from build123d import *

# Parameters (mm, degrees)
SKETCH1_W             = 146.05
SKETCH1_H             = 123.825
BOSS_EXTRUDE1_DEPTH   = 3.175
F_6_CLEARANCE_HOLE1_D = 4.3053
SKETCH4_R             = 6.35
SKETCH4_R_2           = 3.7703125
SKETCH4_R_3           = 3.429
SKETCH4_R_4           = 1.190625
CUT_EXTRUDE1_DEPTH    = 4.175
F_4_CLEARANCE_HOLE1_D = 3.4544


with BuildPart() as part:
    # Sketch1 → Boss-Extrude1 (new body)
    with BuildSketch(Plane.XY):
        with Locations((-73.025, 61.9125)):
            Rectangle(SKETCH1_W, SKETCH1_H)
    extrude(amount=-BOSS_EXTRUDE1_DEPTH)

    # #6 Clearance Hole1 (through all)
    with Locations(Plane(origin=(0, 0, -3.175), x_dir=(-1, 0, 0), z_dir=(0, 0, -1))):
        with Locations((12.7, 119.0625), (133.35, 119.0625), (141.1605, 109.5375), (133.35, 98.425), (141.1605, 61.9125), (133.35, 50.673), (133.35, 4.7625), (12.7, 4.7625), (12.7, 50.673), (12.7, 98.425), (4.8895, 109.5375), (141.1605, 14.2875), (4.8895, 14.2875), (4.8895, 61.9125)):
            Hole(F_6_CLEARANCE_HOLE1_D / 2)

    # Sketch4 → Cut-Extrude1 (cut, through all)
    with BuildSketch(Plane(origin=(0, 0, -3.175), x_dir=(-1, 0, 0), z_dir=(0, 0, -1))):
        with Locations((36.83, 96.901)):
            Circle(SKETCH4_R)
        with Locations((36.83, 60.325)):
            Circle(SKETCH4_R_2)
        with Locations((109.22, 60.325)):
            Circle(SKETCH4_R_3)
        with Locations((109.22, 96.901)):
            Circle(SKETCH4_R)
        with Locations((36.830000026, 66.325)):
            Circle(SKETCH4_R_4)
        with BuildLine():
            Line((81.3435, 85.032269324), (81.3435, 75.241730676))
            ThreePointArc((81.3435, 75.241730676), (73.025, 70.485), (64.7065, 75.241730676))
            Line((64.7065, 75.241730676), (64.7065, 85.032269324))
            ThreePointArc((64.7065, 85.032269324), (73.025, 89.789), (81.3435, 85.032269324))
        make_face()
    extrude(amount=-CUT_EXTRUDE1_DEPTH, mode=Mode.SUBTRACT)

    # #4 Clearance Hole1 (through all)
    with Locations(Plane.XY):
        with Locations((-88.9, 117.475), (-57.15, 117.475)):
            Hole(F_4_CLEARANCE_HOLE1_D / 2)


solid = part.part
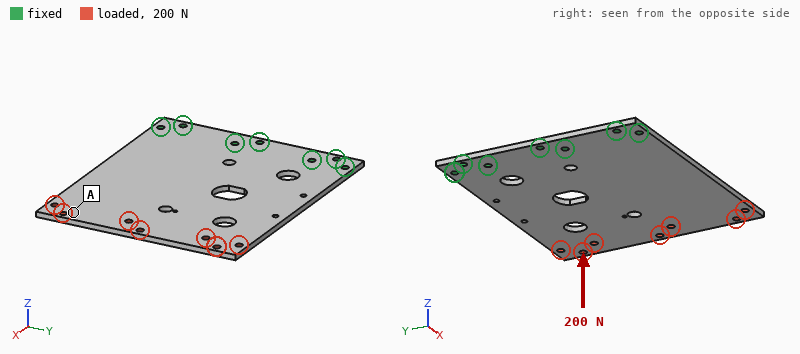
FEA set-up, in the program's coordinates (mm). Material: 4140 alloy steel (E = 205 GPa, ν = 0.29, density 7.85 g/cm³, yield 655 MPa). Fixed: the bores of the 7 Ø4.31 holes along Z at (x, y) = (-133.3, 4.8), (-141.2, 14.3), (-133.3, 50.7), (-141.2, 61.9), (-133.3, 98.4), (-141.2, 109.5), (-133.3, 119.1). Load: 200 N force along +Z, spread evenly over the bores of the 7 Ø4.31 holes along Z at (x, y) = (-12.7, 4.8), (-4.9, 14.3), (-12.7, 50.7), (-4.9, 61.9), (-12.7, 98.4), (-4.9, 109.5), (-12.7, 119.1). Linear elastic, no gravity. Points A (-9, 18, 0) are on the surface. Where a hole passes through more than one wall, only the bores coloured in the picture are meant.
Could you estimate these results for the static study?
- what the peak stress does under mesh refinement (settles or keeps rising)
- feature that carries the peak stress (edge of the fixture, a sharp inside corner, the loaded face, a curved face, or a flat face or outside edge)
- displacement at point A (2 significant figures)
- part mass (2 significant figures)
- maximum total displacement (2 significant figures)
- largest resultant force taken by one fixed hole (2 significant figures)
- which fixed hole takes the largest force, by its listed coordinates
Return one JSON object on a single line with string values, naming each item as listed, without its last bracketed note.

{"what the peak stress does under mesh refinement": "keeps rising", "feature that carries the peak stress": "edge of the fixture", "displacement at point A": "2.0 mm", "part mass": "430 g", "maximum total displacement": "2.3 mm", "largest resultant force taken by one fixed hole": "410 N", "which fixed hole takes the largest force, by its listed coordinates": "(-133.3, 50.7)"}
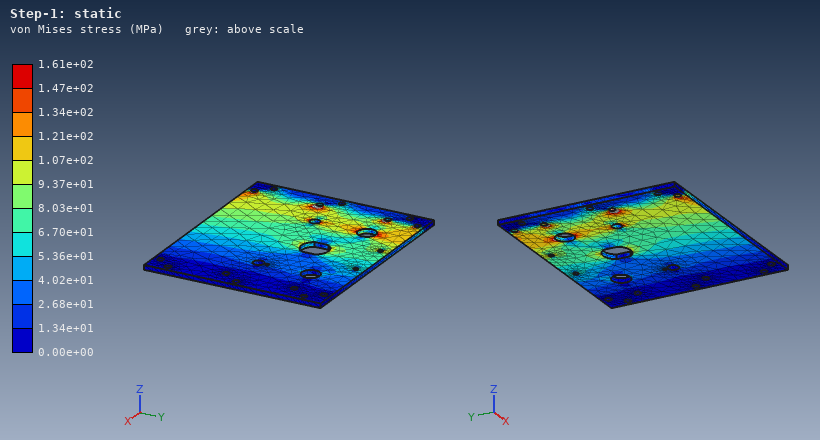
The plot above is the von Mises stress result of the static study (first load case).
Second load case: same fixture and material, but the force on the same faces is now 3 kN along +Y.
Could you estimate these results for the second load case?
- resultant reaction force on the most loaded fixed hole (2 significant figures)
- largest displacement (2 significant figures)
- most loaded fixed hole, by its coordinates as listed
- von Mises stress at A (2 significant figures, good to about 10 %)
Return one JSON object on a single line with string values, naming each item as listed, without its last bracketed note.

{"resultant reaction force on the most loaded fixed hole": "2.3 kN", "largest displacement": "45 µm", "most loaded fixed hole, by its coordinates as listed": "(-133.3, 4.8)", "von Mises stress at A": "14 MPa"}
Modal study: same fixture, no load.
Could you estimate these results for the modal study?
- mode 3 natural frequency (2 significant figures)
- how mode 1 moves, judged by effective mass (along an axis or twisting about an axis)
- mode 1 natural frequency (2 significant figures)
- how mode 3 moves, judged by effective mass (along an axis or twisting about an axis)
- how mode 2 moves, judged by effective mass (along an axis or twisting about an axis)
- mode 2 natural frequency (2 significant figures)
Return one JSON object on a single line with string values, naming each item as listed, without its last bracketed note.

{"mode 3 natural frequency": "900 Hz", "how mode 1 moves, judged by effective mass": "along Z", "mode 1 natural frequency": "150 Hz", "how mode 3 moves, judged by effective mass": "along Z", "how mode 2 moves, judged by effective mass": "twisting about X", "mode 2 natural frequency": "390 Hz"}
